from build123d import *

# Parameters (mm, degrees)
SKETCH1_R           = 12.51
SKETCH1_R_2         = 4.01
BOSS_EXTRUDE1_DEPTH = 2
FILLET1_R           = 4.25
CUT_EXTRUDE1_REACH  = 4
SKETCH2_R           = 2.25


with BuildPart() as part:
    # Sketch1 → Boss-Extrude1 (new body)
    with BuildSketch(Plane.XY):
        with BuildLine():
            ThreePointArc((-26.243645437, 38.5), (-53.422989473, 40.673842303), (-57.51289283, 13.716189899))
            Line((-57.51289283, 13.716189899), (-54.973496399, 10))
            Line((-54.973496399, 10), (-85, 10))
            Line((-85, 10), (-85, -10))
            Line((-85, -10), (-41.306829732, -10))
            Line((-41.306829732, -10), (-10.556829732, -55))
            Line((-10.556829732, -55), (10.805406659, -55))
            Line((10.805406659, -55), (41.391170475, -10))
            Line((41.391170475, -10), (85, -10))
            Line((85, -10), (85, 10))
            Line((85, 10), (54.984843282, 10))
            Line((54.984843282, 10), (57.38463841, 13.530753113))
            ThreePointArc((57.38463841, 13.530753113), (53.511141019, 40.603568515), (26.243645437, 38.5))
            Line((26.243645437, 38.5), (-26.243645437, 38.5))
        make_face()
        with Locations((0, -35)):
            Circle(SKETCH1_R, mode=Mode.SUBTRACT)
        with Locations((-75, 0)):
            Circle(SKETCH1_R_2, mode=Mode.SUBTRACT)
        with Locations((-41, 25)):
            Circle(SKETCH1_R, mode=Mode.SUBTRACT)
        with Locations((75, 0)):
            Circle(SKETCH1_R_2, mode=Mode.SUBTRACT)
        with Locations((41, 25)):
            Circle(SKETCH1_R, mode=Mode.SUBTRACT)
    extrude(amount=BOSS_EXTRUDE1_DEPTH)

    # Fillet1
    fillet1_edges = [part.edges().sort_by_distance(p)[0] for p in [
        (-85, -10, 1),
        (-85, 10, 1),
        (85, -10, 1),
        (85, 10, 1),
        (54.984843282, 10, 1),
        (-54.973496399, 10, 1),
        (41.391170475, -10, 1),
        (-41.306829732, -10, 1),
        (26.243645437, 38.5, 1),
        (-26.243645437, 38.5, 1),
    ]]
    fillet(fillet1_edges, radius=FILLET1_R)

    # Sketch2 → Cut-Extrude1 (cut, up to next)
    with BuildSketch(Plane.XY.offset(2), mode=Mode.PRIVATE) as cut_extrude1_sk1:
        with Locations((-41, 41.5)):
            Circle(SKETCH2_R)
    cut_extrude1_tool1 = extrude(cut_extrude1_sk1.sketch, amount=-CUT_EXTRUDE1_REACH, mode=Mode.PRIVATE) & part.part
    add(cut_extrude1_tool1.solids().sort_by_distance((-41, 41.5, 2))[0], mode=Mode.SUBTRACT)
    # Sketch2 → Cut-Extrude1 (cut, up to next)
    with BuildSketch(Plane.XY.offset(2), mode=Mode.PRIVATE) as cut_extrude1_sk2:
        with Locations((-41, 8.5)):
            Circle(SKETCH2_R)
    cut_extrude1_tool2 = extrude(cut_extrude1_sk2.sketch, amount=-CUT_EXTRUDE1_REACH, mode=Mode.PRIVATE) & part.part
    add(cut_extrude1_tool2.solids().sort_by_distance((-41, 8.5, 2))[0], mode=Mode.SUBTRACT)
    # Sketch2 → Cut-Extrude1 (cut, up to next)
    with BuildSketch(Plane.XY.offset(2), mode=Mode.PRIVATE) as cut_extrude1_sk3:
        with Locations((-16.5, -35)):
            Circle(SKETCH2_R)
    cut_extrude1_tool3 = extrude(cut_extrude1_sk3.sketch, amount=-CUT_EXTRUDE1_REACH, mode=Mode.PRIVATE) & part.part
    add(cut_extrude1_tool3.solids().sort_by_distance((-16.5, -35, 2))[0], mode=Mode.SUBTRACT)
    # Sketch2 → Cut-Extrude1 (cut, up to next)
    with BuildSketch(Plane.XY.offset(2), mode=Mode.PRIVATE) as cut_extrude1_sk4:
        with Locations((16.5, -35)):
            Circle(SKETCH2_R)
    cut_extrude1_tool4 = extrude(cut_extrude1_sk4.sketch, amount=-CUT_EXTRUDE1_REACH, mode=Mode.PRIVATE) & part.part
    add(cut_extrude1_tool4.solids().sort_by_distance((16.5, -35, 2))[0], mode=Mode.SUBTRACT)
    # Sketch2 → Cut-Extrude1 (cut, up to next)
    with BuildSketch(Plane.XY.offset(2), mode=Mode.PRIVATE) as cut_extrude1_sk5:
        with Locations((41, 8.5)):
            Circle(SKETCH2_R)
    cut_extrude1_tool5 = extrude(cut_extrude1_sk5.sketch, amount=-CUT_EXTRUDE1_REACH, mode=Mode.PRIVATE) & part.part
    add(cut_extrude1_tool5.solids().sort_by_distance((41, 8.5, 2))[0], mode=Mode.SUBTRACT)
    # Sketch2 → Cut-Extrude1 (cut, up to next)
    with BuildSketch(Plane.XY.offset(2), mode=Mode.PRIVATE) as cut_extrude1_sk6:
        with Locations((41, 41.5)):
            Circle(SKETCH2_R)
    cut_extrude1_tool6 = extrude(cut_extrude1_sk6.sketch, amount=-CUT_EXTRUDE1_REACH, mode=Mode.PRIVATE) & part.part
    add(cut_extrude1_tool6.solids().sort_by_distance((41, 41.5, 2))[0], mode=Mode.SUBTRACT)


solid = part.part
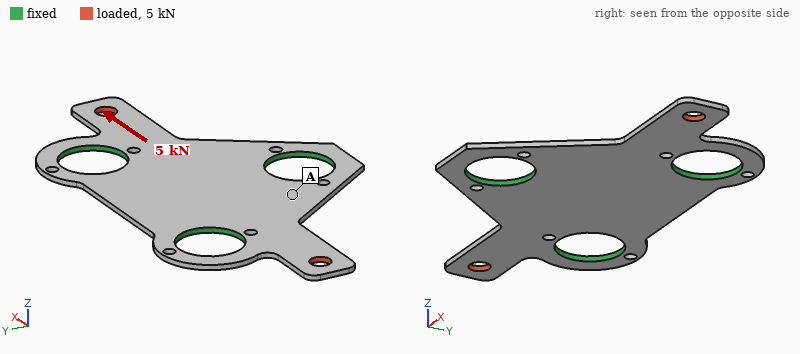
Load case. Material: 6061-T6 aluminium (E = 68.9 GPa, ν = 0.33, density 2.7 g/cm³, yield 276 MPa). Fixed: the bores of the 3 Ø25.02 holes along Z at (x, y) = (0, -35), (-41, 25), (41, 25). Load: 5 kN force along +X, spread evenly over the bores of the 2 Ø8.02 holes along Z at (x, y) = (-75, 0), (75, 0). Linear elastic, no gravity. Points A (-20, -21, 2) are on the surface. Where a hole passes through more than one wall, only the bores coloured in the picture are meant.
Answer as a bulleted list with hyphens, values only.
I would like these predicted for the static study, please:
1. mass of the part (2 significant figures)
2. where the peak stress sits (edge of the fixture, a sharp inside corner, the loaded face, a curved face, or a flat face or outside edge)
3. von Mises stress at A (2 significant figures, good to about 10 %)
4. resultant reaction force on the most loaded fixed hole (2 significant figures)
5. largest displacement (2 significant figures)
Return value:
- 42 g
- the loaded face
- 19 MPa
- 1.8 kN
- 69 µm
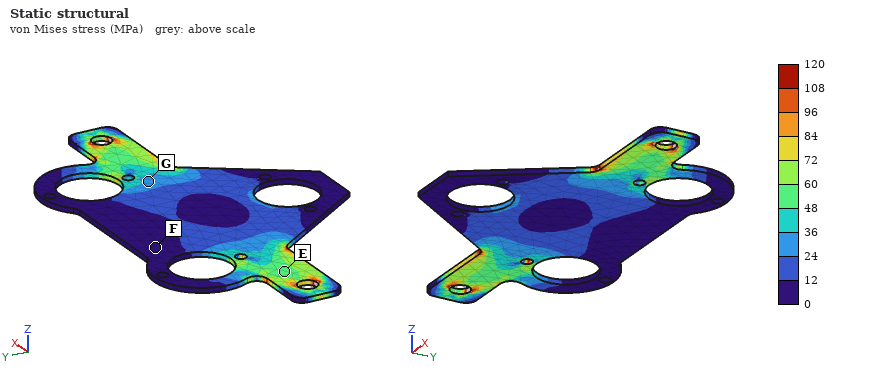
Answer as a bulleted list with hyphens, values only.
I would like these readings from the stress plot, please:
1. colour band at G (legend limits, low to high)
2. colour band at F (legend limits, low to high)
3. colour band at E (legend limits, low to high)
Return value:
- 24 to 36 MPa
- 0 to 12 MPa
- 48 to 60 MPa
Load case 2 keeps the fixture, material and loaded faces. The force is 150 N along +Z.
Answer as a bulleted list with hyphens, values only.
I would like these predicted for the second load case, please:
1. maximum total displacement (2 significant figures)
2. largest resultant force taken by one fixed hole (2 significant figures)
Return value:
- 1.1 mm
- 77 N
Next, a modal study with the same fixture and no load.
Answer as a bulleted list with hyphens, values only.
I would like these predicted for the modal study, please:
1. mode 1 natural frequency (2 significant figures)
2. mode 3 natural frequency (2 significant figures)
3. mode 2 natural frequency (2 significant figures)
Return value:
- 1100 Hz
- 3000 Hz
- 1100 Hz
